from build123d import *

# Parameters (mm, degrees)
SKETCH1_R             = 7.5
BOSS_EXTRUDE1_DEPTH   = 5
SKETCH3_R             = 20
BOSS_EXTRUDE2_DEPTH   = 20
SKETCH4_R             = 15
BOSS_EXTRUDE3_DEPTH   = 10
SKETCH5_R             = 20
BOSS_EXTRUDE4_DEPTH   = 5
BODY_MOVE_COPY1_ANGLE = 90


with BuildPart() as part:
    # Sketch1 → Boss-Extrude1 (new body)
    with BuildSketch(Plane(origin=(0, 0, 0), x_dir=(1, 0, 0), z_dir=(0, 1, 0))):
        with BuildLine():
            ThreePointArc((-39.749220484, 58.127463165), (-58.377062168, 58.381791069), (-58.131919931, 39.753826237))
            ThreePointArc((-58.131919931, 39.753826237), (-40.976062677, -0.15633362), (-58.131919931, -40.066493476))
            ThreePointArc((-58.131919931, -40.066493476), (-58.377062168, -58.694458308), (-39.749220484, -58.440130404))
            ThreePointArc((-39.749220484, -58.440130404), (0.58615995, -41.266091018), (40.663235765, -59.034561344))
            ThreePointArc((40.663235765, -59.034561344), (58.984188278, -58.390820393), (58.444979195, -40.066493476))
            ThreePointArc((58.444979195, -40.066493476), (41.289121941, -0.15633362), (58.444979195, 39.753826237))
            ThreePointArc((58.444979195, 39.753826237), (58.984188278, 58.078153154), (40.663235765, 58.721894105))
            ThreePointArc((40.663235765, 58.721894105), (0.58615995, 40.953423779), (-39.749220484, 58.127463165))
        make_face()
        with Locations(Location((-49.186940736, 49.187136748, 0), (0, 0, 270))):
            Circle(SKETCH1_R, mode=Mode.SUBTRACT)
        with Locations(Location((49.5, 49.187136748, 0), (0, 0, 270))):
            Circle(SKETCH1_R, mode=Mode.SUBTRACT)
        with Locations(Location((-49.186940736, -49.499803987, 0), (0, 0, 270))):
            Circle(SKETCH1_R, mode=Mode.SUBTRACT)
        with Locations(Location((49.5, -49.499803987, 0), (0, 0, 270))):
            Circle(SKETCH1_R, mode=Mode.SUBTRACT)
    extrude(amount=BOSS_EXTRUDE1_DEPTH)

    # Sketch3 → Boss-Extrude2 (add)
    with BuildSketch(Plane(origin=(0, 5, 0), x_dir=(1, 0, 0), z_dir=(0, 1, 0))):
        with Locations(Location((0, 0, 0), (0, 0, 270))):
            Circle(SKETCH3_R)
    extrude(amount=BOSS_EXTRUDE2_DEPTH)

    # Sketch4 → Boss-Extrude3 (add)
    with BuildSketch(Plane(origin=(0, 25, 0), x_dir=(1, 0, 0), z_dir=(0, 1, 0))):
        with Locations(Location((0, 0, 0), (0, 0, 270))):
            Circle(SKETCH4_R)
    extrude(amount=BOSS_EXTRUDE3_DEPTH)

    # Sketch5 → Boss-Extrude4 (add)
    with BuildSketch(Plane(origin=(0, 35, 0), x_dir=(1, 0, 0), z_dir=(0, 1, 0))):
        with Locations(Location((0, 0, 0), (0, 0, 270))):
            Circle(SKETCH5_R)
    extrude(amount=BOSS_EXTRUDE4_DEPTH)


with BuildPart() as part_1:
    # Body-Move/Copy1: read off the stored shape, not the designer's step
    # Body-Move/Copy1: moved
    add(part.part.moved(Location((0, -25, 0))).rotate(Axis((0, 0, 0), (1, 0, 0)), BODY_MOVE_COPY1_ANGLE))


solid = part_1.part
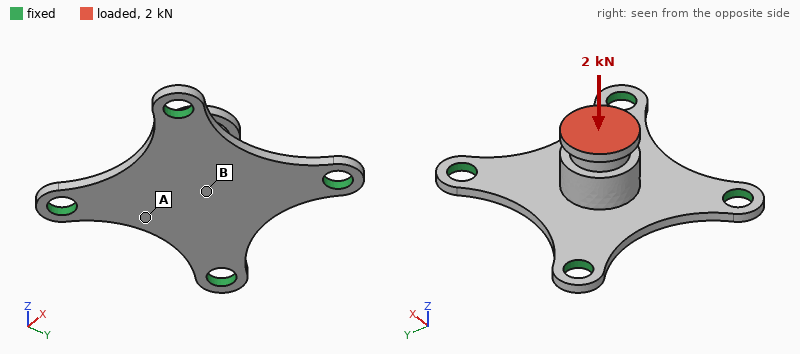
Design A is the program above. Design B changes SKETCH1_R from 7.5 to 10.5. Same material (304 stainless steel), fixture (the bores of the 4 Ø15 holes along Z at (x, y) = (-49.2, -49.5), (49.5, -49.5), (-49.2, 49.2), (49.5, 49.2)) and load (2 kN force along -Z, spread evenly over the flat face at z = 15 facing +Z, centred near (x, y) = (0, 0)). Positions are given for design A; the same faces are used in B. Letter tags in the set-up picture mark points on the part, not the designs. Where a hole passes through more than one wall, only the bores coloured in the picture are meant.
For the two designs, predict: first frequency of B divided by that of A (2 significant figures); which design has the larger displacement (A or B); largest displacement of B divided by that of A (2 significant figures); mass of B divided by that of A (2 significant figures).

1.1
A
0.81
0.96
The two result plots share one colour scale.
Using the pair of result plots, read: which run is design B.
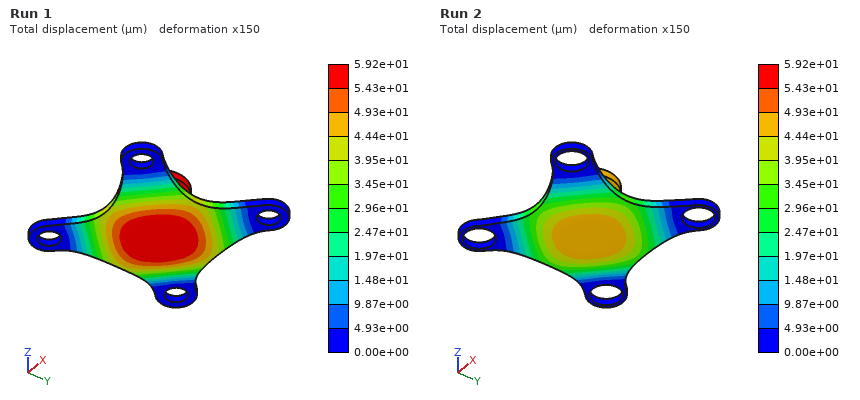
Run 2
